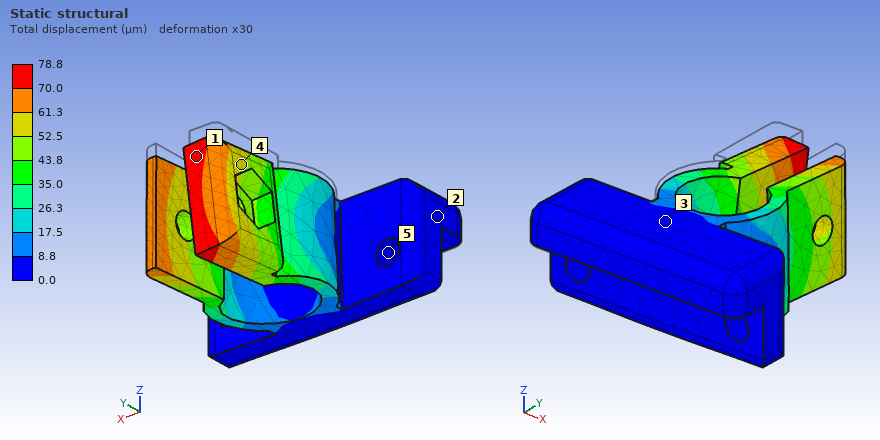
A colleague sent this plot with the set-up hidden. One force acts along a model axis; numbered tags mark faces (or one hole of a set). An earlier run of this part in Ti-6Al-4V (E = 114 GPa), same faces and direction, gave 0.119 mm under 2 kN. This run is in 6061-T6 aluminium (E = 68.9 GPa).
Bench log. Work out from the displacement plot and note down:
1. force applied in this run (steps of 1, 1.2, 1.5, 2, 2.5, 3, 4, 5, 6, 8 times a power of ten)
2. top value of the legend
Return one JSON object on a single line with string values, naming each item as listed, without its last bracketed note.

{"force applied in this run": "800 N", "top value of the legend": "78.8 µm"}
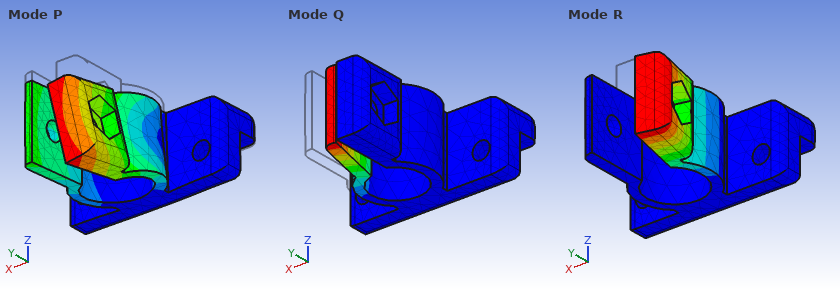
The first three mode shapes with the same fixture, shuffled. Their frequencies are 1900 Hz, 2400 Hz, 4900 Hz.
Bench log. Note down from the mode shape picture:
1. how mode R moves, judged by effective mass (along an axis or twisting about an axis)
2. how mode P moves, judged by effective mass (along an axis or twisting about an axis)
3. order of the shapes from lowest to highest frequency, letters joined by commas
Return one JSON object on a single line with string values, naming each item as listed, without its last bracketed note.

{"how mode R moves, judged by effective mass": "along X", "how mode P moves, judged by effective mass": "along Z", "order of the shapes from lowest to highest frequency, letters joined by commas": "R, Q, P"}
